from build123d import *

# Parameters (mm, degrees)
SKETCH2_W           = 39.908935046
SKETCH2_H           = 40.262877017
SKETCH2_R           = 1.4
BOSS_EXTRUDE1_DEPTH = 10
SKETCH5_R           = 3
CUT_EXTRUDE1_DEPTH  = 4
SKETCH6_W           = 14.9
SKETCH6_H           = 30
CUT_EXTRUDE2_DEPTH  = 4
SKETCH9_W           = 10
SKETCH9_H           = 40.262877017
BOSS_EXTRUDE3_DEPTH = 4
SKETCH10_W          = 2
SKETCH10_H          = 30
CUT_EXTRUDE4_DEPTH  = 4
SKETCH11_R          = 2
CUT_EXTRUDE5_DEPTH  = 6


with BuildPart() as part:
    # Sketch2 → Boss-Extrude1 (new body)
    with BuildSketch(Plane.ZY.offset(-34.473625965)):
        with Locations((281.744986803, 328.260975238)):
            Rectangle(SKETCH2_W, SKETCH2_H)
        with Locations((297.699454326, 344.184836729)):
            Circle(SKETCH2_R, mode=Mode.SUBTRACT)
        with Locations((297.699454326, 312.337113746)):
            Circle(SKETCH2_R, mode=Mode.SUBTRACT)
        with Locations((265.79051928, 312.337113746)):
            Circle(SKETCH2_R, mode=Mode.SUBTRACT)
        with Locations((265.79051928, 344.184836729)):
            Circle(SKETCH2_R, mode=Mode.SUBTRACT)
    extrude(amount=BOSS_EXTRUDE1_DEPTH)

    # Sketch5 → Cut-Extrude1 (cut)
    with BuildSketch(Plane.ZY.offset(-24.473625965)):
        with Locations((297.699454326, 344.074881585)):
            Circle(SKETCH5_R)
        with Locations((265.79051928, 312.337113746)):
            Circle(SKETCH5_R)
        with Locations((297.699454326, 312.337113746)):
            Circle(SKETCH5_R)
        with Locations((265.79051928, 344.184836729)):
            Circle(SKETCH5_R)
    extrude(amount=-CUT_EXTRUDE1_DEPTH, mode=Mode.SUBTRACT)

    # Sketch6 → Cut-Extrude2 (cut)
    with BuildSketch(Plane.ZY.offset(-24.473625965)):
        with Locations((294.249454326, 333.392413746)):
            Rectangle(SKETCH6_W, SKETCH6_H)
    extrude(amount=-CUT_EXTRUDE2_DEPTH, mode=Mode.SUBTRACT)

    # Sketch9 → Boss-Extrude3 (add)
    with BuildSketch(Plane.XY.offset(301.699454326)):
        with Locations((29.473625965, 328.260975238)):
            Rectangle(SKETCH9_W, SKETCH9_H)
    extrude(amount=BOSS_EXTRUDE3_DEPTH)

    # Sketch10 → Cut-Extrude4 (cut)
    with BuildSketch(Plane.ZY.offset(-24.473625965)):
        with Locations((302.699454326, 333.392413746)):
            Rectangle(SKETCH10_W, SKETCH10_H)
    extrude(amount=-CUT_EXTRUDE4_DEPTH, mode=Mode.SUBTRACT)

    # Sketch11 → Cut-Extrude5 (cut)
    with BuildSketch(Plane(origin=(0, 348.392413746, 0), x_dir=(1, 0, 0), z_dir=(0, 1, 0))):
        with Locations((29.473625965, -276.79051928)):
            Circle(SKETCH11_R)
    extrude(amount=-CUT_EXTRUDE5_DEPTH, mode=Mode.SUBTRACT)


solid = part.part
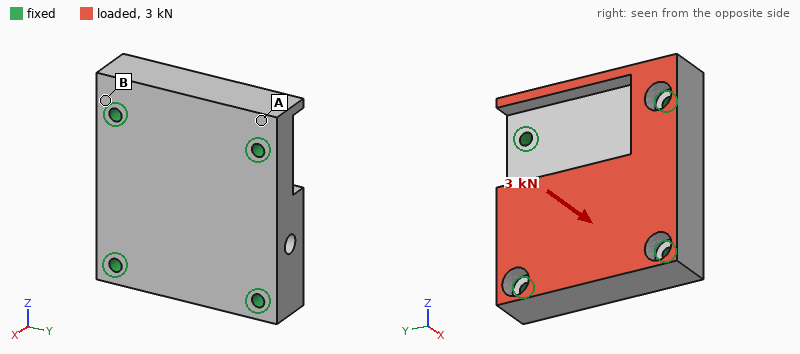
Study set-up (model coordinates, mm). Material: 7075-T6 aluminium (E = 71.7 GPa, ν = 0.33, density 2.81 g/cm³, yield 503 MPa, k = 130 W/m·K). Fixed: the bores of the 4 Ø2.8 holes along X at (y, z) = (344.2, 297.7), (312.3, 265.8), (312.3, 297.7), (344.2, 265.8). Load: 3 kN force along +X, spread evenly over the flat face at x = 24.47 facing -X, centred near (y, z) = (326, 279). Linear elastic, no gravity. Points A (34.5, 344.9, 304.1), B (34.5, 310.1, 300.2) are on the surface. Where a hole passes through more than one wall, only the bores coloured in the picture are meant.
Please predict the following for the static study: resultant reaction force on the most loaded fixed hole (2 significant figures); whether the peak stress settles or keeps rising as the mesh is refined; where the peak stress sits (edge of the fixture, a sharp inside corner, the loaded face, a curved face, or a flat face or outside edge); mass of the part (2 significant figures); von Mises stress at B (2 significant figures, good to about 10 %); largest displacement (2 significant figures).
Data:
930 N
keeps rising
edge of the fixture
42 g
10 MPa
7.0 µm
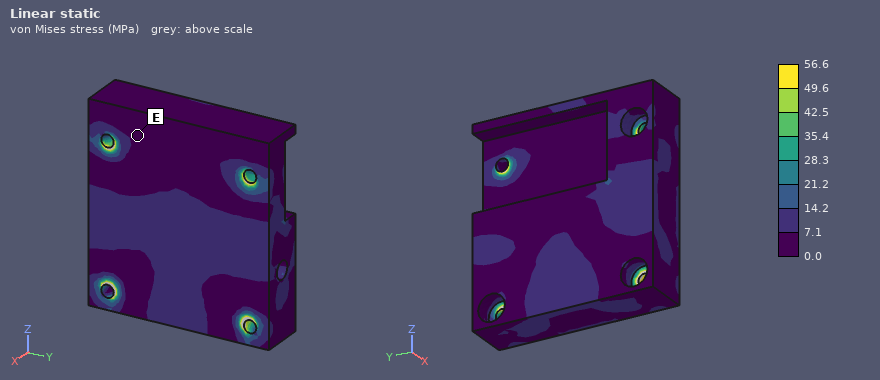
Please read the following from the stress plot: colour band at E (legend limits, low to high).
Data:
0.0 to 7.1 MPa
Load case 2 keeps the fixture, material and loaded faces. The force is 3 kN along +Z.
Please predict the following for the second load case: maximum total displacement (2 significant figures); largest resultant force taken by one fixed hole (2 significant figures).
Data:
7.7 µm
970 N
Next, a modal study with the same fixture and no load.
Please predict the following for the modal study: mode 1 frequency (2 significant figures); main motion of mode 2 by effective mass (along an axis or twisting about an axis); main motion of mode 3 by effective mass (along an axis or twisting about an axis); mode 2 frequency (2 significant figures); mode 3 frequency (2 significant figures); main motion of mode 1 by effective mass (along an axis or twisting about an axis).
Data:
19 kHz
twisting about Y
twisting about Z
25 kHz
28 kHz
along X
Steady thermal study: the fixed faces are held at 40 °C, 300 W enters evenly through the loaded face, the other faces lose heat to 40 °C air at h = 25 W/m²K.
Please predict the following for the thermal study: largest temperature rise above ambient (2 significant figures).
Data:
61 K
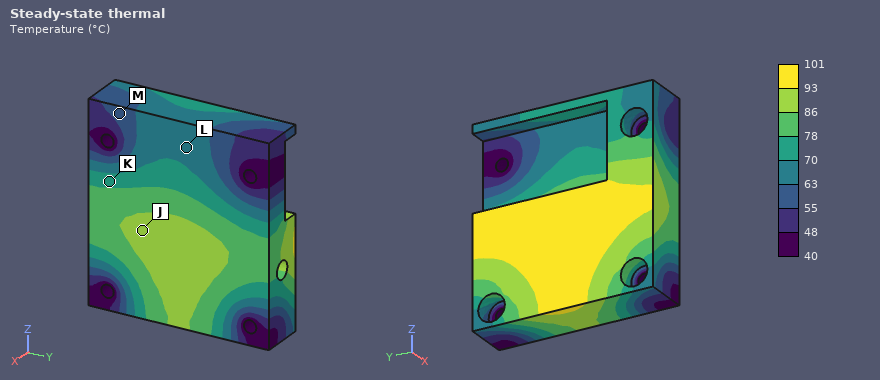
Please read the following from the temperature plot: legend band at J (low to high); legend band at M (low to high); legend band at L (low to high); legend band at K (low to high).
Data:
86 to 93 °C
55 to 63 °C
63 to 70 °C
70 to 78 °C
